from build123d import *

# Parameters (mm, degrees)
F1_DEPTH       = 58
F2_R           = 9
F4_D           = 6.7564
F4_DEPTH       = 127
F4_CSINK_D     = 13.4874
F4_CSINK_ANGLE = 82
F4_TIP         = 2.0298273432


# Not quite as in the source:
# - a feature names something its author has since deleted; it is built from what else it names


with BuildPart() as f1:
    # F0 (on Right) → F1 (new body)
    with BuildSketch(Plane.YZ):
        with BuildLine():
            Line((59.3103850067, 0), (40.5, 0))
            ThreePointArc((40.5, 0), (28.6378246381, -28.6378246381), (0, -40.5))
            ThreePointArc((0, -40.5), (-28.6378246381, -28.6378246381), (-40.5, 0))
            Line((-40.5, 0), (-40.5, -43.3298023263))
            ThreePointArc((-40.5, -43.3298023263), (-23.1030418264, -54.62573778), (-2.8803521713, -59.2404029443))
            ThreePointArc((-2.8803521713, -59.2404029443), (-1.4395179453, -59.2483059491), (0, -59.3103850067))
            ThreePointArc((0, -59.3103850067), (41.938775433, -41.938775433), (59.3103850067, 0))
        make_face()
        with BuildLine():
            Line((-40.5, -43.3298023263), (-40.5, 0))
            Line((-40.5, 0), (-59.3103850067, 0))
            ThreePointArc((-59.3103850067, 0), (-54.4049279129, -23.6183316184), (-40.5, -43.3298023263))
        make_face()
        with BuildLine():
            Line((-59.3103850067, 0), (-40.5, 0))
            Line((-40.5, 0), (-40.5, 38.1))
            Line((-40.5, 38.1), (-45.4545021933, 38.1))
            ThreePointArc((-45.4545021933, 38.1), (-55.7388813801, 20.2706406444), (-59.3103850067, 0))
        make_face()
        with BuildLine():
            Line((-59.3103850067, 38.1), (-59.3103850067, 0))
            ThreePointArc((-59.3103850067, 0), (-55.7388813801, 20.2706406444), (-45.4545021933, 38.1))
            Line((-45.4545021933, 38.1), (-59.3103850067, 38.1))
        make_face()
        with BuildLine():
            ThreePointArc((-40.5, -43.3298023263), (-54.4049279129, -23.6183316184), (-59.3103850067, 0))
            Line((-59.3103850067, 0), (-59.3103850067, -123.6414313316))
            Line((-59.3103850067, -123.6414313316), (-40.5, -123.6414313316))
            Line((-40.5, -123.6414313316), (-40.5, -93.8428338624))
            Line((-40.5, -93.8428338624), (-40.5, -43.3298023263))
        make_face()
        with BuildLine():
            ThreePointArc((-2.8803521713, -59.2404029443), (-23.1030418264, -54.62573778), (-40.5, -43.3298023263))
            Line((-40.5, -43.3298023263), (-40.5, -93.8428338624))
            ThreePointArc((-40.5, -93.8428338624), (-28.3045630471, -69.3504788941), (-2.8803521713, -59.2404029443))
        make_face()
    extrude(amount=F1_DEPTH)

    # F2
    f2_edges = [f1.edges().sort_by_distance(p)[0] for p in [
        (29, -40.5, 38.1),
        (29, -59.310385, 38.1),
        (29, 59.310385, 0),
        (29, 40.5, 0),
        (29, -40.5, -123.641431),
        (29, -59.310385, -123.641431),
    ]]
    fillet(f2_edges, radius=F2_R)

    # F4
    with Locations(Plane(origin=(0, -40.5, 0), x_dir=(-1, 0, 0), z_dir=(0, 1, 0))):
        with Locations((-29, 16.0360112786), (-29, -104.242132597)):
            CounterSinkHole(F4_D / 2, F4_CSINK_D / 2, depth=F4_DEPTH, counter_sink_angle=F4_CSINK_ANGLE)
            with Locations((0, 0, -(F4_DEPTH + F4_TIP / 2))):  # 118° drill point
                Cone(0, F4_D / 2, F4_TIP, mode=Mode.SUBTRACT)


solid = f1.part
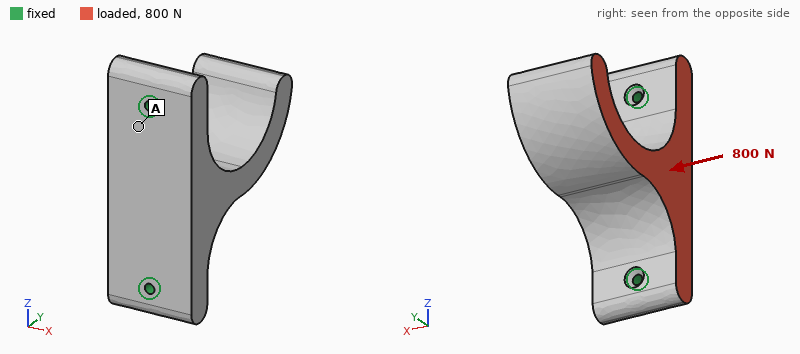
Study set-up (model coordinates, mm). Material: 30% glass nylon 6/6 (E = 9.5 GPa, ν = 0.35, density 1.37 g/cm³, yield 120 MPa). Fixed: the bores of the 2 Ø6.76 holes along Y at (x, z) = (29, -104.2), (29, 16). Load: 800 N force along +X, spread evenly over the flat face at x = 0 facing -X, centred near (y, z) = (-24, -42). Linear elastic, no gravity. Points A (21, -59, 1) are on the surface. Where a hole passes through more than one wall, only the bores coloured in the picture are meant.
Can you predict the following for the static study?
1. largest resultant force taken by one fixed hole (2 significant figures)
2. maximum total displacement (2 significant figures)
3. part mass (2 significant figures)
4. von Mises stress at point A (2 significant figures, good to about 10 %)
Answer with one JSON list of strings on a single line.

["410 N", "0.19 mm", "460 g", "1.4 MPa"]
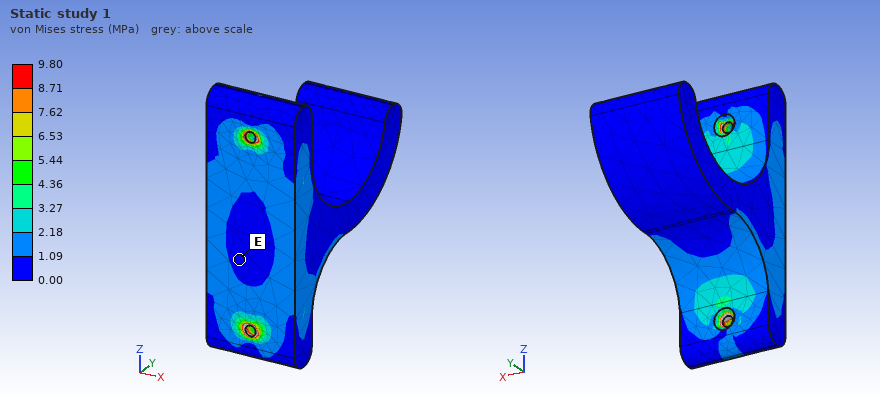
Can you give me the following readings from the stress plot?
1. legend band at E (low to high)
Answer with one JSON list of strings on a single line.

["0.00 to 1.09 MPa"]
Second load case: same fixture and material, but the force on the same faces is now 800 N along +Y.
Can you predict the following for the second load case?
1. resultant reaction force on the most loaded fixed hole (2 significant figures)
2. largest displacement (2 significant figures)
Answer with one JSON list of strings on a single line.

["470 N", "0.18 mm"]
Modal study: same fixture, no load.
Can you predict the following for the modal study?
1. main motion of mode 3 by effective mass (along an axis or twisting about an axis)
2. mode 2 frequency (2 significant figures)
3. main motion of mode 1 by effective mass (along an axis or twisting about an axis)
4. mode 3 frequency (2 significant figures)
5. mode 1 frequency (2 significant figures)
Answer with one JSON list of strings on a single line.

["along Y", "820 Hz", "along X", "1900 Hz", "580 Hz"]
